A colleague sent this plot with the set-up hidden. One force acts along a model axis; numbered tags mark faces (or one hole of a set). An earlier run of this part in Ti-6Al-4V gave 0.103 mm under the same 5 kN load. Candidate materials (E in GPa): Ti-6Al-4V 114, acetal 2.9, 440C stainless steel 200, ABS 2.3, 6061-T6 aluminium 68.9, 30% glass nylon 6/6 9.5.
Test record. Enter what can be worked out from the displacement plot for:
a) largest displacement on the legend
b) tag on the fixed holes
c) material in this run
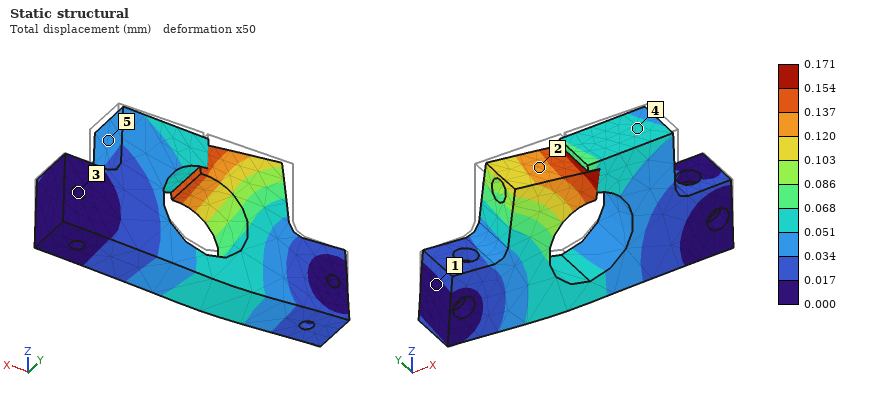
0.171 mm
3
6061-T6 aluminium
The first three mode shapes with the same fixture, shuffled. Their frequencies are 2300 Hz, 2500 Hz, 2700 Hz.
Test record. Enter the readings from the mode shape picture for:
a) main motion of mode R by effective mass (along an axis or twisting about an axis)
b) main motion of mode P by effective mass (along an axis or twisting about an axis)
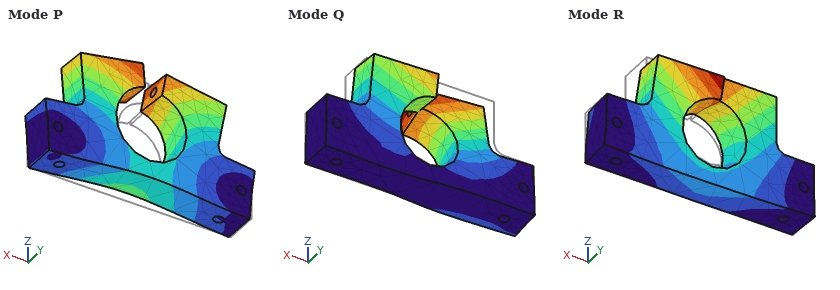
along Y
along Z
